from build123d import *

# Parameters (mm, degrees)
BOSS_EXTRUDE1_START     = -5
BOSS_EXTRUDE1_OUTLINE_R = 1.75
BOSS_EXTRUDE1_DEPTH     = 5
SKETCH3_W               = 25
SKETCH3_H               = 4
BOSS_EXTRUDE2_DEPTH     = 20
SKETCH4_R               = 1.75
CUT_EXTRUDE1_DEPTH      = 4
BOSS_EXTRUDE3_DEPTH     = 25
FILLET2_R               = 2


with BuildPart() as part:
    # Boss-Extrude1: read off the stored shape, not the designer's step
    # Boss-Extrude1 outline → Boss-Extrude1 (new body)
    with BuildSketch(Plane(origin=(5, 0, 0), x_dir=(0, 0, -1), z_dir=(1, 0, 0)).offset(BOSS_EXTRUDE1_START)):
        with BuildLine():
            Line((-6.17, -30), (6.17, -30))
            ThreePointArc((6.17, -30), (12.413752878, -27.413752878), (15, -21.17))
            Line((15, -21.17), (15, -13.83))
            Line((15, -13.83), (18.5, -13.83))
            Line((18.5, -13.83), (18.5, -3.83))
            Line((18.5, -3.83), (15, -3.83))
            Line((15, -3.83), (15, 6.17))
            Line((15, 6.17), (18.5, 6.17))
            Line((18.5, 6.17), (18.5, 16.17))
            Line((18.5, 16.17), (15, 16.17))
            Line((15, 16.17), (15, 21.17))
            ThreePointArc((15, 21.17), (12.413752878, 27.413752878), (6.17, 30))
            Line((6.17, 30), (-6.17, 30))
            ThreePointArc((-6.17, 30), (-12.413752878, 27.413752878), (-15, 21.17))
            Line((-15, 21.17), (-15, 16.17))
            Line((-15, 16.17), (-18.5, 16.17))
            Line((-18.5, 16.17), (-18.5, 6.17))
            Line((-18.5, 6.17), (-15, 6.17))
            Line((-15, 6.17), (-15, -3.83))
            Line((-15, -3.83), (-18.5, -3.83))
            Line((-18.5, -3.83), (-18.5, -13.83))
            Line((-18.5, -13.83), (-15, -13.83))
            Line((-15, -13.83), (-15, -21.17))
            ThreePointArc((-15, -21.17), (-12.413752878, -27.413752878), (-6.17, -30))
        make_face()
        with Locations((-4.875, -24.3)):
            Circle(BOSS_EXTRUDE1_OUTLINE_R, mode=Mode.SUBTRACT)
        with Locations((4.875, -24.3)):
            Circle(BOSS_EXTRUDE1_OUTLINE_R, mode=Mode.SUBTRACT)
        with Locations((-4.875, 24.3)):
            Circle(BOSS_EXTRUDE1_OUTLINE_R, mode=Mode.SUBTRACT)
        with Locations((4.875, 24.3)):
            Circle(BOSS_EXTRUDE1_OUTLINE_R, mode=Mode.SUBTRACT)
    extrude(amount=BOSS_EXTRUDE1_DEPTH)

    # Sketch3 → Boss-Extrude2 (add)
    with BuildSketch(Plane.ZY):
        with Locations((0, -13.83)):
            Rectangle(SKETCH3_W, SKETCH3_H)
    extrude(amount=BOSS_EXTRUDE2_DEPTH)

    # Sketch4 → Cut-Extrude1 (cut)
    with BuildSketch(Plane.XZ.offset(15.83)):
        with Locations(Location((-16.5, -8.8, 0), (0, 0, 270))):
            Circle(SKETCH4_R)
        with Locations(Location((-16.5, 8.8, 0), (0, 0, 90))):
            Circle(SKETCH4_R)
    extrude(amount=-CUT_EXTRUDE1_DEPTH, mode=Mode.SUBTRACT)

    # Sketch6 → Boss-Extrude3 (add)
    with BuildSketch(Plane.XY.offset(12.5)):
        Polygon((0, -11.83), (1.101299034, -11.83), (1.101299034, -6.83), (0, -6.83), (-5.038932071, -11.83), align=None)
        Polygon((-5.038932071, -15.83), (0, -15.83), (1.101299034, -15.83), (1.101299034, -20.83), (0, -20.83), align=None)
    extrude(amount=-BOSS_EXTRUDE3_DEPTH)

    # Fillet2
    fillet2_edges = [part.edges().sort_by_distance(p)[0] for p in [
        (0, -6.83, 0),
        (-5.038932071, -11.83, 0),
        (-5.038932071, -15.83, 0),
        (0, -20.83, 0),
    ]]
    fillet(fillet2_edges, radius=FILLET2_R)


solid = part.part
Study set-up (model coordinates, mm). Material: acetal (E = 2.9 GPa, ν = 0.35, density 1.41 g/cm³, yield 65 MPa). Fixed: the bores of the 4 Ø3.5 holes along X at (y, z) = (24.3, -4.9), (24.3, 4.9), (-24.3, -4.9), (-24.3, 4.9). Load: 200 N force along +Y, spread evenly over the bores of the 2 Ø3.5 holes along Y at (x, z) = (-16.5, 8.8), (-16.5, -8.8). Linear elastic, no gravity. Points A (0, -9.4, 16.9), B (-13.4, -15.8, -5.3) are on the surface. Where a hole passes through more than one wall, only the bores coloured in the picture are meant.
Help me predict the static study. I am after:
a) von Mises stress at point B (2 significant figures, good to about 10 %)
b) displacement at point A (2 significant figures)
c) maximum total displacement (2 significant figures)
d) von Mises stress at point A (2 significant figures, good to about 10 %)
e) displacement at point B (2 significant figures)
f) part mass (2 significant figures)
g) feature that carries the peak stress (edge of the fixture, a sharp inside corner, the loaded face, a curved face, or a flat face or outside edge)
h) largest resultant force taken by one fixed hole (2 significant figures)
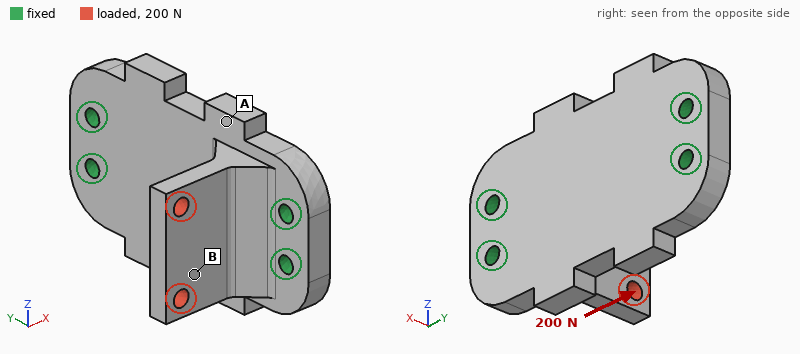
9.3 MPa
0.12 mm
0.77 mm
2.8 MPa
0.39 mm
17 g
a curved face
90 N
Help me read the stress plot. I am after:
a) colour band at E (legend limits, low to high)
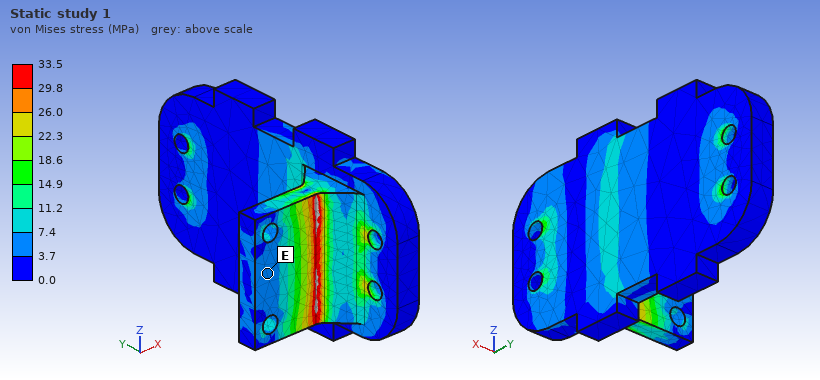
3.7 to 7.4 MPa
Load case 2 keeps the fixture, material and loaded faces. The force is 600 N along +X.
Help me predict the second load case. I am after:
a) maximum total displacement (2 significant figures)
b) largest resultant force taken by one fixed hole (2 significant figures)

0.32 mm
260 N
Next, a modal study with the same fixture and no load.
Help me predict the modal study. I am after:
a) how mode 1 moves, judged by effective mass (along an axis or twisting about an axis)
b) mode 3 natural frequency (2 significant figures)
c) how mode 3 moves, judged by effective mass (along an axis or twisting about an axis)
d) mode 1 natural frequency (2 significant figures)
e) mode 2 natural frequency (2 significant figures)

along X
3900 Hz
along X
2200 Hz
2800 Hz
